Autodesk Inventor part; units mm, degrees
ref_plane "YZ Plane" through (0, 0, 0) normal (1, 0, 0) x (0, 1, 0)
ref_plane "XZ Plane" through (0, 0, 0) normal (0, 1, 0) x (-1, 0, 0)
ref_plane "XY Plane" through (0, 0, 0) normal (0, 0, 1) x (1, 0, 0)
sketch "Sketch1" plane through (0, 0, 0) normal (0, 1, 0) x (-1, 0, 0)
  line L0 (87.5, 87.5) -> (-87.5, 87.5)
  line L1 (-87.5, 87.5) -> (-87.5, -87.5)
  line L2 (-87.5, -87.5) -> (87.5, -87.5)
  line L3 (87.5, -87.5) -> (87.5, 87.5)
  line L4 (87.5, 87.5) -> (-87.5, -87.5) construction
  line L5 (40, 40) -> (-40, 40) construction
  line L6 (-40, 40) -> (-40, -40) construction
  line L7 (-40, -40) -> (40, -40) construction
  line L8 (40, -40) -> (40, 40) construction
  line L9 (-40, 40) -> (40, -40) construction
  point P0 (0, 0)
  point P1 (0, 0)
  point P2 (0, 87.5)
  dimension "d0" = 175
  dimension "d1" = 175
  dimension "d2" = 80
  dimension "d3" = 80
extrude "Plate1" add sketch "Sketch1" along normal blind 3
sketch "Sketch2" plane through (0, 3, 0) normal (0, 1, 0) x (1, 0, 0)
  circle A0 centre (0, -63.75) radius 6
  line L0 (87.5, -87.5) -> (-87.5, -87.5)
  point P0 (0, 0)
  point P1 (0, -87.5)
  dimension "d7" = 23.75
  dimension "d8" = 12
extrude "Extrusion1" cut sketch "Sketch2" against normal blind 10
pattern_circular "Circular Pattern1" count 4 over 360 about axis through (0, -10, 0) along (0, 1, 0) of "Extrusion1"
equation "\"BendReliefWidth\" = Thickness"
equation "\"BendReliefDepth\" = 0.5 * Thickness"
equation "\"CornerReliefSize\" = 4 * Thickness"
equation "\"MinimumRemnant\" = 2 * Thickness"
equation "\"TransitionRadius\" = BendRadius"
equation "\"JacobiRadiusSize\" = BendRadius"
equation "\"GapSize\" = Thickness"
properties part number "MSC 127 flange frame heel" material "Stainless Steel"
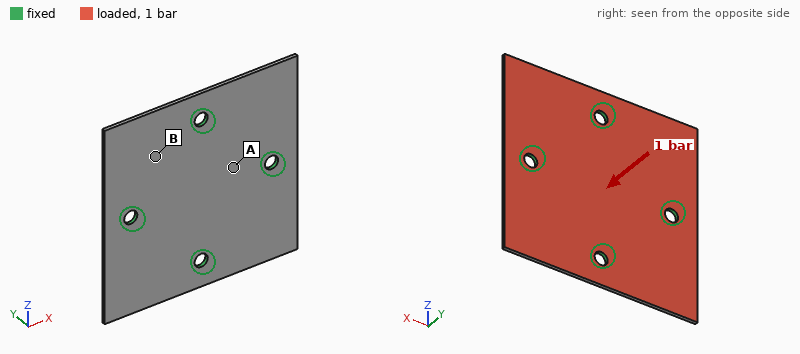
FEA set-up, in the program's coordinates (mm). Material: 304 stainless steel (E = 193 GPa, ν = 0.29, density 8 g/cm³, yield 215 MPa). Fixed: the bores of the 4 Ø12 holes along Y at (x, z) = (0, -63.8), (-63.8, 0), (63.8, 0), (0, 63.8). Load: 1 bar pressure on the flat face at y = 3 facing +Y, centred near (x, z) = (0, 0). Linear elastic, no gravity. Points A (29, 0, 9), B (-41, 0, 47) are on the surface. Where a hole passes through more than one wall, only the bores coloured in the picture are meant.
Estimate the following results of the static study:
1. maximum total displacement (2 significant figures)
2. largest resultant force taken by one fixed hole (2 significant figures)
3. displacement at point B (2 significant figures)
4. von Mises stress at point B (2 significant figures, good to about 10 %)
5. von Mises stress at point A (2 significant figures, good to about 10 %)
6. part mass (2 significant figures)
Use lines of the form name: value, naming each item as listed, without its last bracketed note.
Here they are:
maximum total displacement: 0.47 mm
largest resultant force taken by one fixed hole: 750 N
displacement at point B: 0.090 mm
von Mises stress at point B: 45 MPa
von Mises stress at point A: 19 MPa
part mass: 720 g
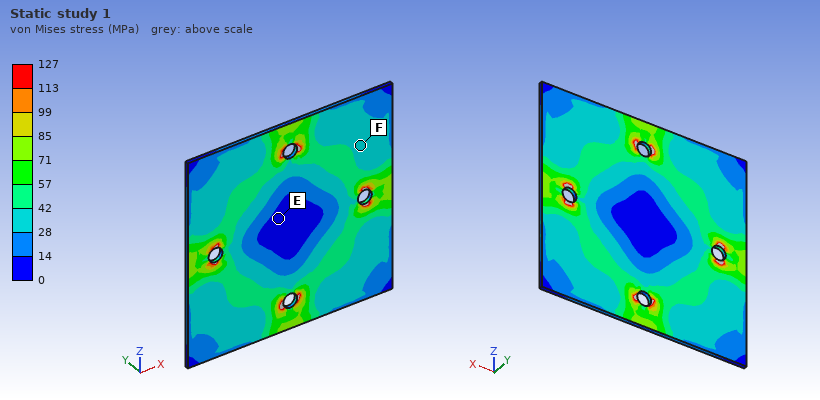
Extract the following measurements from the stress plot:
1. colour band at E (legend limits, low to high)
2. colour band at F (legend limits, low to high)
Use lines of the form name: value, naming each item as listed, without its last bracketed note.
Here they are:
colour band at E: 0 to 14 MPa
colour band at F: 28 to 42 MPa
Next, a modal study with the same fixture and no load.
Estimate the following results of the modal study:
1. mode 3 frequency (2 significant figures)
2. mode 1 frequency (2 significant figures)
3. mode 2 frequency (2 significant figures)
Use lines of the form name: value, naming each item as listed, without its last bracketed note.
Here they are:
mode 3 frequency: 660 Hz
mode 1 frequency: 650 Hz
mode 2 frequency: 660 Hz
